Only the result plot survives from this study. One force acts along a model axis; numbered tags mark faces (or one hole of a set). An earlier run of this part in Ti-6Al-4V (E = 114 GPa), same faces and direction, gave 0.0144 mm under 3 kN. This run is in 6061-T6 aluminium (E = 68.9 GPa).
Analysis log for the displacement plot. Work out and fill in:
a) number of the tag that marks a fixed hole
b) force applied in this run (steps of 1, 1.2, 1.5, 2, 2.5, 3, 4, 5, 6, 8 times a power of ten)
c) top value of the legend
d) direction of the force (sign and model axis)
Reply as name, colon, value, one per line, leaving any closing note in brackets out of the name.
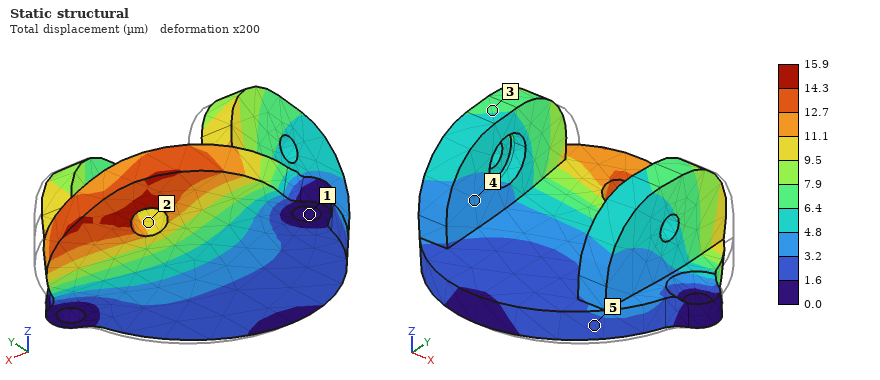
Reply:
number of the tag that marks a fixed hole: 1
force applied in this run: 2 kN
top value of the legend: 15.9 µm
direction of the force: -X
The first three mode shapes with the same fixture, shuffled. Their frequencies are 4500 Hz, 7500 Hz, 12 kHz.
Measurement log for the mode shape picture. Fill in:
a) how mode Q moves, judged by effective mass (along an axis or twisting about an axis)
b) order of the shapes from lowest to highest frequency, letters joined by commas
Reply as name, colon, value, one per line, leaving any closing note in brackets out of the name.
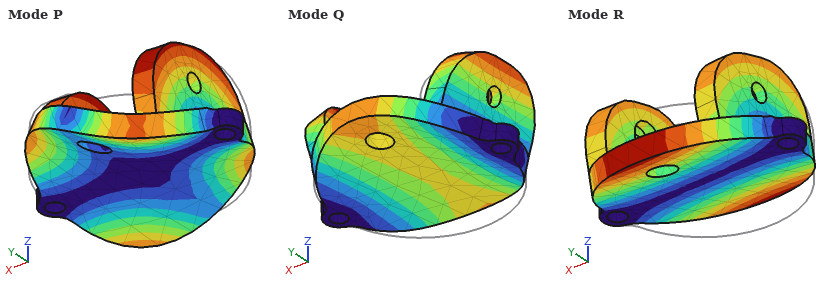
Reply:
how mode Q moves, judged by effective mass: along Z
order of the shapes from lowest to highest frequency, letters joined by commas: R, Q, P
